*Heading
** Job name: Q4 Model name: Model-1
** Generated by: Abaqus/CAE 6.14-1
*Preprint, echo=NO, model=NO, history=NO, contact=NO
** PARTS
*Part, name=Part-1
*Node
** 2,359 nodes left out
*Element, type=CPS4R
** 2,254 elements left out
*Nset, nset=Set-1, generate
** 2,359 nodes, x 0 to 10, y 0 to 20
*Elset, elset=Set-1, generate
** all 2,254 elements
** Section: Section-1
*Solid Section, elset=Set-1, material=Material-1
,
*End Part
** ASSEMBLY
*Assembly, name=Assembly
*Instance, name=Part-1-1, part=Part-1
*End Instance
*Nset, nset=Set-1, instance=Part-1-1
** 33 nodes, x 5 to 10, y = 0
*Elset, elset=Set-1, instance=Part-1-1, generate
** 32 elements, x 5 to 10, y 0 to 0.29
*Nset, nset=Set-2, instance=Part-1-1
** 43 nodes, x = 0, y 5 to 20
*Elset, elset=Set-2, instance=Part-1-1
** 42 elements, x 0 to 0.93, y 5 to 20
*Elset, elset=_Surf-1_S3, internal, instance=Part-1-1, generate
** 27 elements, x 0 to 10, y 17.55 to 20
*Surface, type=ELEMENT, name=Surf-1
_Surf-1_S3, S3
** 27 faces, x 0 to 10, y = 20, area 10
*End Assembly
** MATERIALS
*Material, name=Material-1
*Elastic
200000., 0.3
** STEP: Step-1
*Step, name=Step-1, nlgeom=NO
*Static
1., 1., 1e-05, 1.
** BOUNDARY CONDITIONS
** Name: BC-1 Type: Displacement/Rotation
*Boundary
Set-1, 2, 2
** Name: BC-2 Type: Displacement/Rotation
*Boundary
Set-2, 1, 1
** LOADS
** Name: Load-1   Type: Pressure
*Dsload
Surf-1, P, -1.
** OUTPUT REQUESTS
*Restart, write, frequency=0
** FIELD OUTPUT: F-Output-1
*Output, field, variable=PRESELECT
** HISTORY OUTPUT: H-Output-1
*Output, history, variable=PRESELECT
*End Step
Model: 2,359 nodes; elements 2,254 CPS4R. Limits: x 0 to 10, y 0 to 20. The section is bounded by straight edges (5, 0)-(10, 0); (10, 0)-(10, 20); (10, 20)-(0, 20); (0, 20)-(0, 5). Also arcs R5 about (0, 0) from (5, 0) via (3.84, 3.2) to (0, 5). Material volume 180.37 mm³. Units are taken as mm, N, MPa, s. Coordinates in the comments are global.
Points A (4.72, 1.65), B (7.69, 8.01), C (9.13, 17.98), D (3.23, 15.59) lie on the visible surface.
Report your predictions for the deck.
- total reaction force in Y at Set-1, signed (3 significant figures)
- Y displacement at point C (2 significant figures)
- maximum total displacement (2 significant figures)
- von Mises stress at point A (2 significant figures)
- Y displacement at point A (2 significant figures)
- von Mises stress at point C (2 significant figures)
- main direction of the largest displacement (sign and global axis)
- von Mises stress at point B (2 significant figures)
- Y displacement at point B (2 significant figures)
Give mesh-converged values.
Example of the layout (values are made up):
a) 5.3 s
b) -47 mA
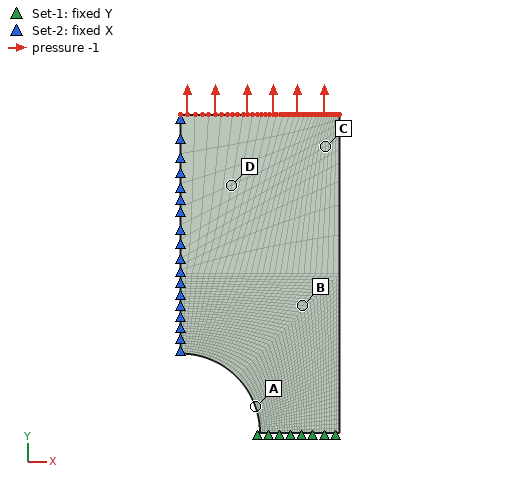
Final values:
a) -10.0 N
b) 1.3e-04 mm
c) 1.5e-04 mm
d) 3.4 MPa
e) 3.6e-05 mm
f) 1.0 MPa
g) +Y
h) 1.5 MPa
i) 6.6e-05 mm
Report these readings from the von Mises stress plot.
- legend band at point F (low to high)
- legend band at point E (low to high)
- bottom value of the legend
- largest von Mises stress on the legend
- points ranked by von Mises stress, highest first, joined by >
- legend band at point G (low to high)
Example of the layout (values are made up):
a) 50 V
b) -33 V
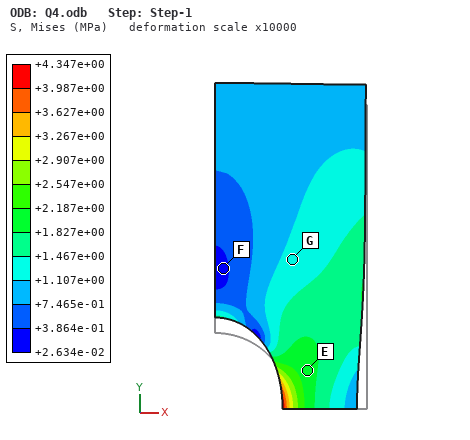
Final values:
a) +2.634e-02 to +3.864e-01 MPa
b) +1.827e+00 to +2.187e+00 MPa
c) +2.634e-02 MPa
d) +4.347e+00 MPa
e) E > G > F
f) +1.107e+00 to +1.467e+00 MPa
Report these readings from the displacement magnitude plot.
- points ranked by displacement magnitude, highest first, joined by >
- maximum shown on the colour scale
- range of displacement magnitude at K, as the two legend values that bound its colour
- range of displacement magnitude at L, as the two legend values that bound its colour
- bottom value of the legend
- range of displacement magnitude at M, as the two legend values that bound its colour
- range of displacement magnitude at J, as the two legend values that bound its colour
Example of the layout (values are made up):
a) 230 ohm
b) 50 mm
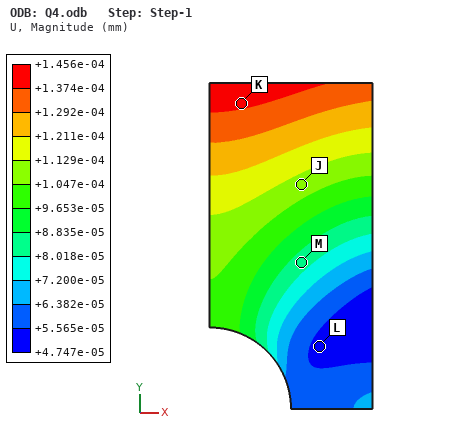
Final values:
a) K > J > M > L
b) +1.456e-04 mm
c) +1.374e-04 to +1.456e-04 mm
d) +4.747e-05 to +5.565e-05 mm
e) +4.747e-05 mm
f) +8.018e-05 to +8.835e-05 mm
g) +1.047e-04 to +1.129e-04 mm
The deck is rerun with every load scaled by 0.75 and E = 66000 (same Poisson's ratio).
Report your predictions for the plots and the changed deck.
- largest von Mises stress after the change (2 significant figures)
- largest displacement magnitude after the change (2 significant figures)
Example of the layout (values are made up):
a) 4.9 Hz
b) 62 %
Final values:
a) 3.3 MPa
b) 3.3e-04 mm
